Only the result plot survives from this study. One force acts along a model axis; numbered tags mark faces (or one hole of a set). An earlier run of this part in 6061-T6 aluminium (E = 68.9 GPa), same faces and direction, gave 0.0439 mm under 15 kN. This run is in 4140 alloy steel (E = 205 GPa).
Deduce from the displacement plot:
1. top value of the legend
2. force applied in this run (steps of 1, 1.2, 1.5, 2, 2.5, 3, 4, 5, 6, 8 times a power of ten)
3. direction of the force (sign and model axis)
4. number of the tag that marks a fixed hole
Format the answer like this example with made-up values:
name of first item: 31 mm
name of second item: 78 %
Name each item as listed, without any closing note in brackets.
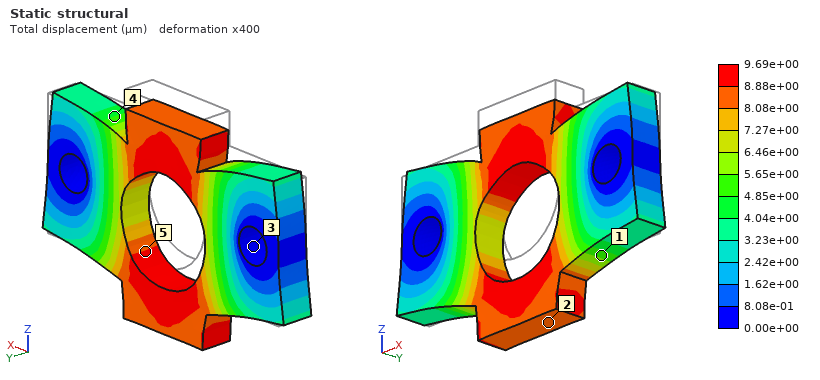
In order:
top value of the legend: 9.69e+00 µm
force applied in this run: 10 kN
direction of the force: -Z
number of the tag that marks a fixed hole: 3
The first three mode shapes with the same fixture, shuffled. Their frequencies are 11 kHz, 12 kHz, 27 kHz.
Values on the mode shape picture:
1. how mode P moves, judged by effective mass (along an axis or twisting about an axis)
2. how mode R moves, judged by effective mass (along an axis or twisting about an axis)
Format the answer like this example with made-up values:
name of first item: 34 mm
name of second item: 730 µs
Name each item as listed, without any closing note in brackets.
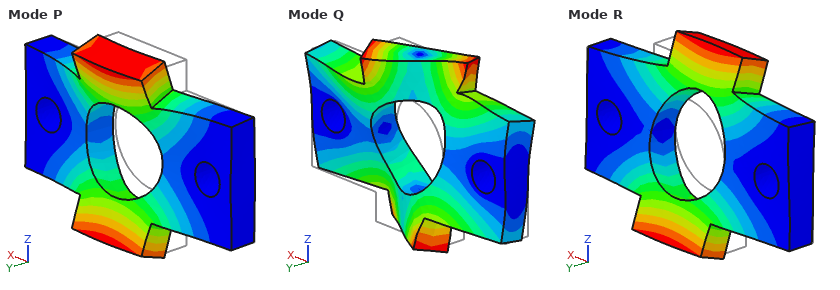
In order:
how mode P moves, judged by effective mass: along Y
how mode R moves, judged by effective mass: twisting about X
